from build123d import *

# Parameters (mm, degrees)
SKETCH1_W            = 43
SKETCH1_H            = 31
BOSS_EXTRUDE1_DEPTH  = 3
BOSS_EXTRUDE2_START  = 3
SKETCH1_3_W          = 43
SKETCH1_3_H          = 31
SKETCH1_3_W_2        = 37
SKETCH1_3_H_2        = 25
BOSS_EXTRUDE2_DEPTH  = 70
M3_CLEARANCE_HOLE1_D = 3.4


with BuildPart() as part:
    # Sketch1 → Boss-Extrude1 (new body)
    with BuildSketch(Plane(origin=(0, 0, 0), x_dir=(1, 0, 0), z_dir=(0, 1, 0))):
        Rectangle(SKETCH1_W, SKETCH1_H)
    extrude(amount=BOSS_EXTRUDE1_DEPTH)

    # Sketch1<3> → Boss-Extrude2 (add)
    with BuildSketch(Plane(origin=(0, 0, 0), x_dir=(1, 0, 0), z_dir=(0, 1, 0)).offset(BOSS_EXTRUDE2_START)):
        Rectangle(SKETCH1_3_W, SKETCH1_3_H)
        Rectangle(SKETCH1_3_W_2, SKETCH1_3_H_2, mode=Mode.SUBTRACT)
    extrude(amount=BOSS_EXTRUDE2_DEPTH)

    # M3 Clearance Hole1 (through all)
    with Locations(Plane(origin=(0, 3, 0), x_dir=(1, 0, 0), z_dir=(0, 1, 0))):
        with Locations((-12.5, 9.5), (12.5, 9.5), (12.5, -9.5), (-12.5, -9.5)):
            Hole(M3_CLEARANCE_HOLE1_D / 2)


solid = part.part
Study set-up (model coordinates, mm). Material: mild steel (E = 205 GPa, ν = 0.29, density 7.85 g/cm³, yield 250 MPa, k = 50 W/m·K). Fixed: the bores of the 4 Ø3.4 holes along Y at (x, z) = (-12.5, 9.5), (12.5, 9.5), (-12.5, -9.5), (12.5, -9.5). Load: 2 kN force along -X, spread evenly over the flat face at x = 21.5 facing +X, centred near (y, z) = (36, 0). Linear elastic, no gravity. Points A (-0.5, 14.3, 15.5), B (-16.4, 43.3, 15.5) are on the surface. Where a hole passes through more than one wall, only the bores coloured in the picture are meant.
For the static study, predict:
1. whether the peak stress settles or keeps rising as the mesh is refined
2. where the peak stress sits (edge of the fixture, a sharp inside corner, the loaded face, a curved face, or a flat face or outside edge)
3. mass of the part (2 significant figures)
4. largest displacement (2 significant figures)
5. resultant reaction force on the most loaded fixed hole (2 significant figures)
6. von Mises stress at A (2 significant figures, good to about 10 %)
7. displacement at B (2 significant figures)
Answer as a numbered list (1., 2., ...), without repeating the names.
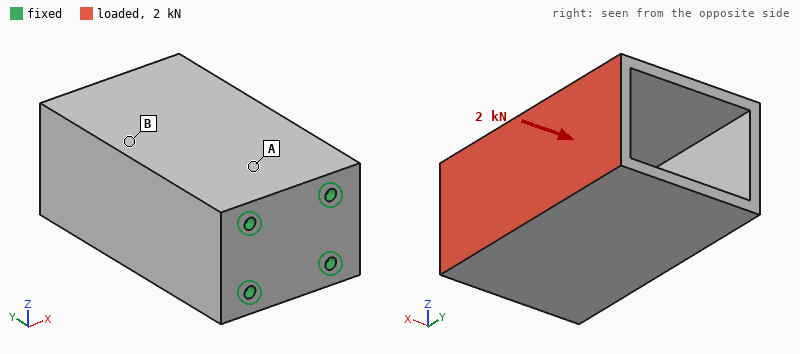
1. keeps rising
2. edge of the fixture
3. 250 g
4. 40 µm
5. 1.4 kN
6. 26 MPa
7. 19 µm
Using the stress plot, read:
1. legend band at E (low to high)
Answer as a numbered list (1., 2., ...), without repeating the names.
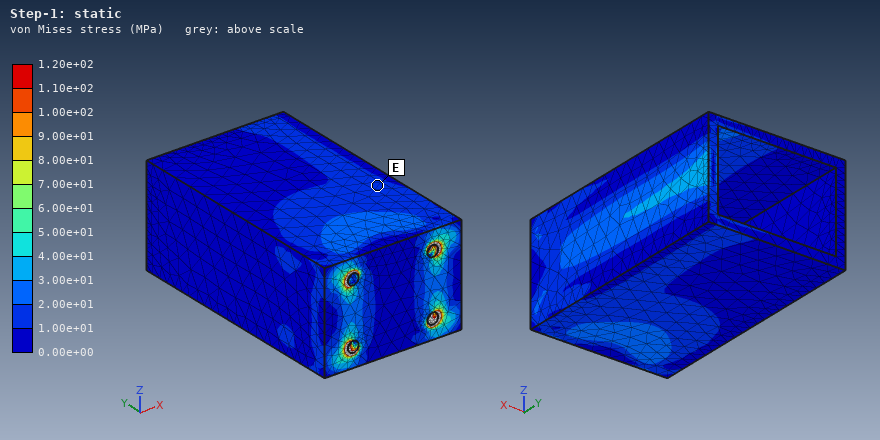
1. 1.00e+01 to 2.00e+01 MPa
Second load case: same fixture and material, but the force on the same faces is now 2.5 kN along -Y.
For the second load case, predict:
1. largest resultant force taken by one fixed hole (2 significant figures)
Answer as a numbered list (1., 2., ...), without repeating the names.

1. 1.6 kN
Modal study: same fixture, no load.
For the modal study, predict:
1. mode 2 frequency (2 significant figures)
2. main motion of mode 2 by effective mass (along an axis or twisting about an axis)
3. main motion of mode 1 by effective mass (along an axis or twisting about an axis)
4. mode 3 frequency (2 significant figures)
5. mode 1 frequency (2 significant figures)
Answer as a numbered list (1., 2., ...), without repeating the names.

1. 3100 Hz
2. along X
3. along Z
4. 4200 Hz
5. 2600 Hz
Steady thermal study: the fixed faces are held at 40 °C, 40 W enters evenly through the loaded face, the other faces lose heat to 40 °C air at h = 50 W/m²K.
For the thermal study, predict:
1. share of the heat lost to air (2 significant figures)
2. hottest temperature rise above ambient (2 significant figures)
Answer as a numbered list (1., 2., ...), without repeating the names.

1. 53 %
2. 57 K
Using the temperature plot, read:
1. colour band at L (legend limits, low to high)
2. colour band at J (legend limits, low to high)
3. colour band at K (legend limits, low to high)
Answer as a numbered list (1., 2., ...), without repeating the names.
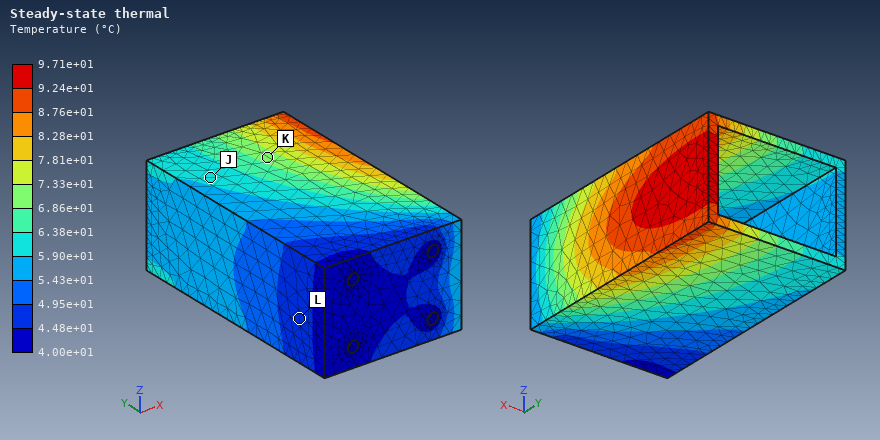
1. 4.48e+01 to 4.95e+01 °C
2. 5.90e+01 to 6.38e+01 °C
3. 6.86e+01 to 7.33e+01 °C
